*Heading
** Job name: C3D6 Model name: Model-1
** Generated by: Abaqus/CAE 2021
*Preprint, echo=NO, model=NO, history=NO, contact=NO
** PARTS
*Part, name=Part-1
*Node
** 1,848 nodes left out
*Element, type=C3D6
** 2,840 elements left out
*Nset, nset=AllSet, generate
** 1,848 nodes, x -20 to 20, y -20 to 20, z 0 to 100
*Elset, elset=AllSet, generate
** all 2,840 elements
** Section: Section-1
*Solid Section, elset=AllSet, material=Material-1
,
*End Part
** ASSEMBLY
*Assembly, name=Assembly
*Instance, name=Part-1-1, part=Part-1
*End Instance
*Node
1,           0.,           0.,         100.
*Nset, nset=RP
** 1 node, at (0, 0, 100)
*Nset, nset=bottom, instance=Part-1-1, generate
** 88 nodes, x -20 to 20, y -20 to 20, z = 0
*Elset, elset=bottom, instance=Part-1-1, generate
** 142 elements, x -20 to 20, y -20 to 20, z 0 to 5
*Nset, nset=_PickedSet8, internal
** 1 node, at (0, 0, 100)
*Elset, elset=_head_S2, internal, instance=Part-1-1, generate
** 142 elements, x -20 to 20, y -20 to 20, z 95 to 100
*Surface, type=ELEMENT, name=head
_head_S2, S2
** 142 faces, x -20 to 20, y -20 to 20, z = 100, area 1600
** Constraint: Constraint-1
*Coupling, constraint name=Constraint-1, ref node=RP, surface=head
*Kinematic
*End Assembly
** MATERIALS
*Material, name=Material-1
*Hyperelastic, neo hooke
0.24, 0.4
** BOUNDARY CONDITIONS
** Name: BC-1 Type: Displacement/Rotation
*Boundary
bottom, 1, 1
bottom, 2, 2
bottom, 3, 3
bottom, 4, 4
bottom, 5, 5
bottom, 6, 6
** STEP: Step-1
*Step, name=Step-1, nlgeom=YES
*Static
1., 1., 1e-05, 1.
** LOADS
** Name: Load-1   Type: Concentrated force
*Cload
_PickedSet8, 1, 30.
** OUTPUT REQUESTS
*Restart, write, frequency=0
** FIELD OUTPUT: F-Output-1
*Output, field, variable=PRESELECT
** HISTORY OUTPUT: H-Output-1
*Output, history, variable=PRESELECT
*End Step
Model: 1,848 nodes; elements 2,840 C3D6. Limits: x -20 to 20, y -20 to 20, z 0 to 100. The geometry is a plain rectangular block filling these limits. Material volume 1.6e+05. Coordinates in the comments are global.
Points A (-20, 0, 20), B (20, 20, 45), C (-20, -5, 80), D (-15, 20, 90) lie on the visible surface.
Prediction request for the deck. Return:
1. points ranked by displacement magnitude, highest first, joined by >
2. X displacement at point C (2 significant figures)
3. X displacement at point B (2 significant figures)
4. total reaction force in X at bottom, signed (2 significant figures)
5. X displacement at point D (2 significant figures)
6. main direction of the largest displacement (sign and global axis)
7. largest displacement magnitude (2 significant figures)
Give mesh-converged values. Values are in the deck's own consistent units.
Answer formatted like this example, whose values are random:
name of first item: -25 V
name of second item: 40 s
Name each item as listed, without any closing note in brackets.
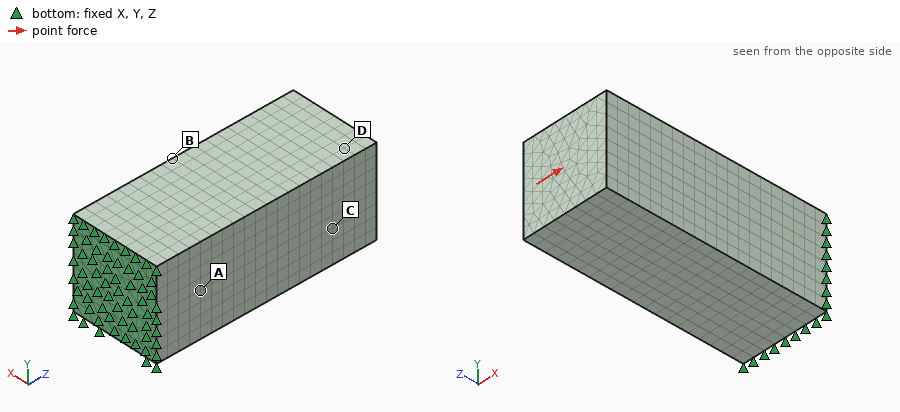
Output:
points ranked by displacement magnitude, highest first, joined by >: D > C > B > A
X displacement at point C: 26
X displacement at point B: 8.2
total reaction force in X at bottom, signed: -30
X displacement at point D: 30
main direction of the largest displacement: +X
largest displacement magnitude: 35
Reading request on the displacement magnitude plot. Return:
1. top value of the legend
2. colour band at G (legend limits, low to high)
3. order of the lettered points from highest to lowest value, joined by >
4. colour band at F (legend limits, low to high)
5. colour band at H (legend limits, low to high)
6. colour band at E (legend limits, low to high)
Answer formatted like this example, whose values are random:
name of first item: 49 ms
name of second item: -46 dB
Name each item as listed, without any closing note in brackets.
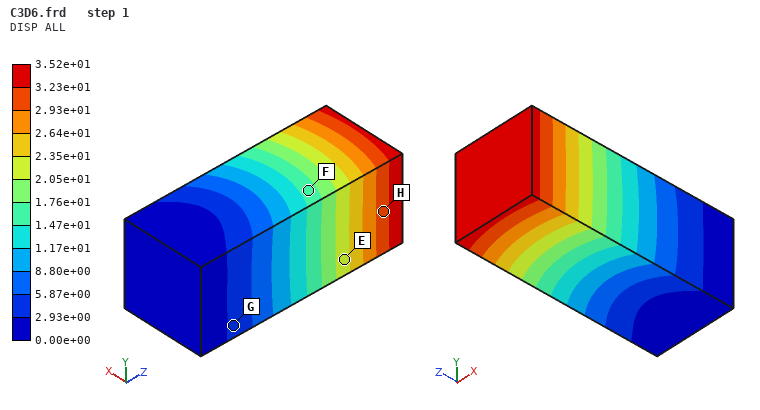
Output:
top value of the legend: 3.52e+01
colour band at G: 2.93e+00 to 5.87e+00
order of the lettered points from highest to lowest value, joined by >: H > E > F > G
colour band at F: 1.47e+01 to 1.76e+01
colour band at H: 2.93e+01 to 3.23e+01
colour band at E: 2.05e+01 to 2.35e+01
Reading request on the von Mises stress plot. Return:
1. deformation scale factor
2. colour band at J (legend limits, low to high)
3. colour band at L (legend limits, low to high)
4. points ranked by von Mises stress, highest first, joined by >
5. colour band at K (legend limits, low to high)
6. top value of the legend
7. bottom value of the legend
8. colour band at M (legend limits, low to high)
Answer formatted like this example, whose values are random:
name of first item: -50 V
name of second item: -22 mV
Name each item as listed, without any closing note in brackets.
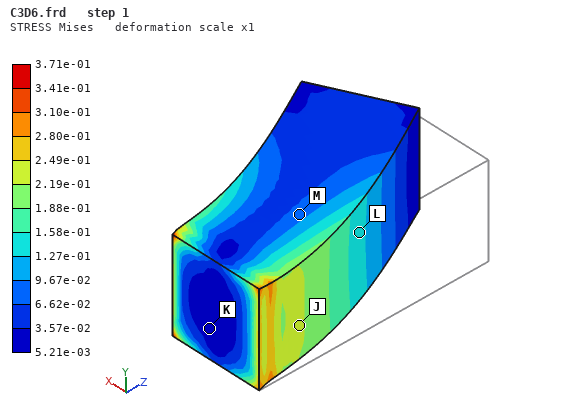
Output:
deformation scale factor: 1
colour band at J: 2.19e-01 to 2.49e-01
colour band at L: 1.27e-01 to 1.58e-01
points ranked by von Mises stress, highest first, joined by >: J > L > M > K
colour band at K: 5.21e-03 to 3.57e-02
top value of the legend: 3.71e-01
bottom value of the legend: 5.21e-03
colour band at M: 6.62e-02 to 9.67e-02
